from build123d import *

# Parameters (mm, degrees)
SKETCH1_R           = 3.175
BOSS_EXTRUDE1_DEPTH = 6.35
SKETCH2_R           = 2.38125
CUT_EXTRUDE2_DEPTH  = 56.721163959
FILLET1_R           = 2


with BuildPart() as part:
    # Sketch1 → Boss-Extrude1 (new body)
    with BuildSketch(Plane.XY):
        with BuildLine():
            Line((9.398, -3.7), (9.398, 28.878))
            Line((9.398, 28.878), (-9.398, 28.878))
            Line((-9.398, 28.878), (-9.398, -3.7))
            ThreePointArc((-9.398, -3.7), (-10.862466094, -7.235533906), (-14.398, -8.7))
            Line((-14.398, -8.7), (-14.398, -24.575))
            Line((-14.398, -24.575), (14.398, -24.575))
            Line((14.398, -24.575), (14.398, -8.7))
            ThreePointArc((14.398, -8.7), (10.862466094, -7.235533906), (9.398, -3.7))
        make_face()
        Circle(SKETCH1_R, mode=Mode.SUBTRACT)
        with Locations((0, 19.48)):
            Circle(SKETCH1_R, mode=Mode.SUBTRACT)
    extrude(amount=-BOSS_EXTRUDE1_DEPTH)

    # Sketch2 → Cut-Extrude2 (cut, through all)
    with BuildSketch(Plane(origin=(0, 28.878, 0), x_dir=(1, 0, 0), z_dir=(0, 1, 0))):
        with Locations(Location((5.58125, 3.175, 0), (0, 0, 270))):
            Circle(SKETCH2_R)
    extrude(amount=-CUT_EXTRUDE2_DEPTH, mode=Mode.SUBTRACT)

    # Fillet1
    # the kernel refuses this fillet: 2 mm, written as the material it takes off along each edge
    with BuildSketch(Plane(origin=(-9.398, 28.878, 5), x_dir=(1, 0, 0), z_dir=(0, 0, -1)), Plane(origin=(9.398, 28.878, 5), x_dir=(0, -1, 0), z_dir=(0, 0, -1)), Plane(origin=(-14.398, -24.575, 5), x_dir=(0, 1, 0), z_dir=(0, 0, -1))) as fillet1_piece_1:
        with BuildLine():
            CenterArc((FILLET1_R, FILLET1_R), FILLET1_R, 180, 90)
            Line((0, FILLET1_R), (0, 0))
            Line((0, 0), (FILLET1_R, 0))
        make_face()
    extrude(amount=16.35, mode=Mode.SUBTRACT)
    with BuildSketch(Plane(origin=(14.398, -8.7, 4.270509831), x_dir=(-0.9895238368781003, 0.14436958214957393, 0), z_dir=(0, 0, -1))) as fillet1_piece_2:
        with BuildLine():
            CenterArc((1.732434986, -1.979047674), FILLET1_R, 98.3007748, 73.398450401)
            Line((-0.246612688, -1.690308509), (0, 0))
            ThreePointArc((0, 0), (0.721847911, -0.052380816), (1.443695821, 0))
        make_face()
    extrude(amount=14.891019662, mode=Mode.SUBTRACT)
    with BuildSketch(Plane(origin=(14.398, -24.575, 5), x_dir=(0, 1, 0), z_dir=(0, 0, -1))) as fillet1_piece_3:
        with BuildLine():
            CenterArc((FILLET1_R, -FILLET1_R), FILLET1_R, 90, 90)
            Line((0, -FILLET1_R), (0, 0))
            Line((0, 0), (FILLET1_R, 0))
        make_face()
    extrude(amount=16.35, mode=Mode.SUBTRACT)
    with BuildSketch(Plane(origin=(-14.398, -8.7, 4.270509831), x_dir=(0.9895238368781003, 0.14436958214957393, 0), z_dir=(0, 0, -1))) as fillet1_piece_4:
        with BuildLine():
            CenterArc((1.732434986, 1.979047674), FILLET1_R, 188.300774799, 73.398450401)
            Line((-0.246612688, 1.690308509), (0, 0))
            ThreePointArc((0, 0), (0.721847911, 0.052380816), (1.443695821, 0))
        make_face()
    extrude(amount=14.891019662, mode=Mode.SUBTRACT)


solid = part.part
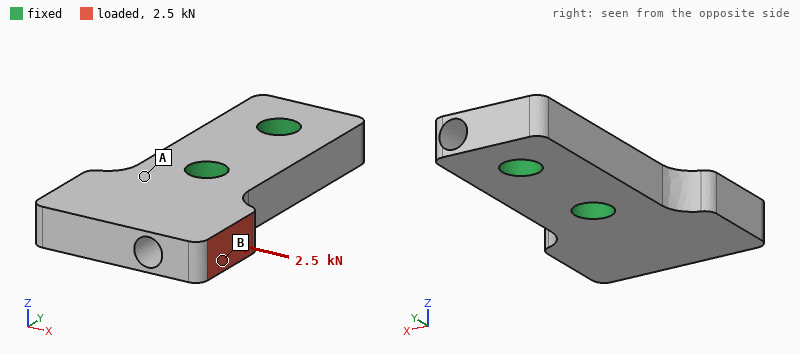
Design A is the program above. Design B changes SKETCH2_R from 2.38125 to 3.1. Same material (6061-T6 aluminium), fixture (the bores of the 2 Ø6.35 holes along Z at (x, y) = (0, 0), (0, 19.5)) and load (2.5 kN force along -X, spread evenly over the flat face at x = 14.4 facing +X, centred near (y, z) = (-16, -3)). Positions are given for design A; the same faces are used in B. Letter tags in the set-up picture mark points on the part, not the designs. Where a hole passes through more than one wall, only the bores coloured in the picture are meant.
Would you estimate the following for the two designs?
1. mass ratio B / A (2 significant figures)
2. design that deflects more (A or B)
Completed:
0.89
B
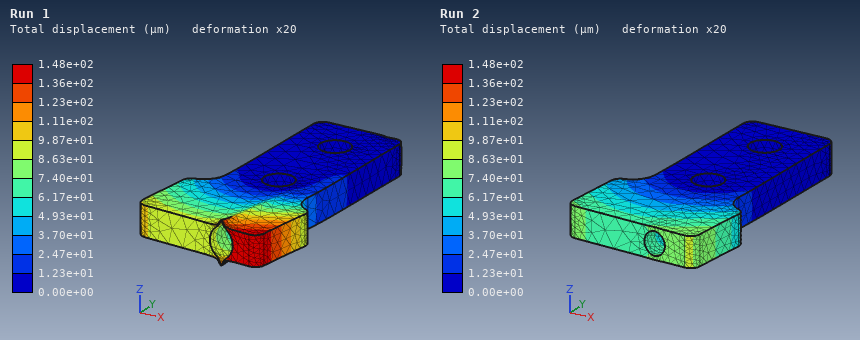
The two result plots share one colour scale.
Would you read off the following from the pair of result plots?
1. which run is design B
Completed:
Run 1
